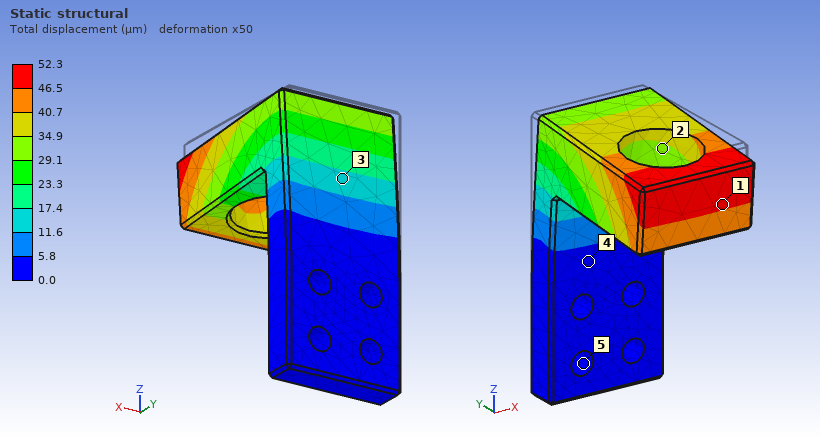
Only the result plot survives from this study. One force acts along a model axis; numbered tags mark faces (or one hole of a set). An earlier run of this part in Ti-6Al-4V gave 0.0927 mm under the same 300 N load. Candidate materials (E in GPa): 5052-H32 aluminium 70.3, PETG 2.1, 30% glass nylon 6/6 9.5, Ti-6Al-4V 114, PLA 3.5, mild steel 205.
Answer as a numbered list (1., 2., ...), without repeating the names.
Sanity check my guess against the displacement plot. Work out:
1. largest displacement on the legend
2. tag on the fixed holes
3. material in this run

1. 52.3 µm
2. 5
3. mild steel
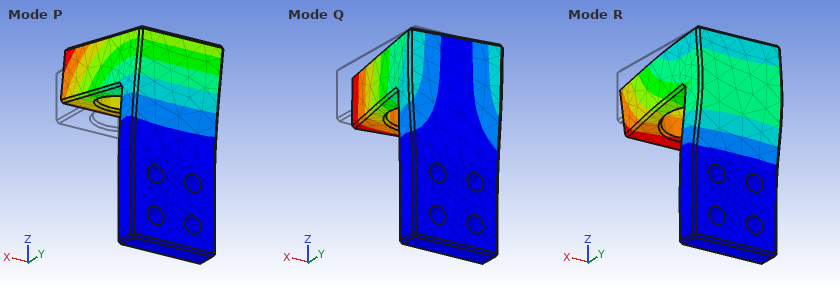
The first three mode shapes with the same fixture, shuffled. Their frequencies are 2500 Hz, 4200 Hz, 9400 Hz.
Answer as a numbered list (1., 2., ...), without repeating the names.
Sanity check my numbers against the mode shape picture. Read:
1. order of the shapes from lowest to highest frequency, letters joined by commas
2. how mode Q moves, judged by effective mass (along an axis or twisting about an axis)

1. P, Q, R
2. along X
